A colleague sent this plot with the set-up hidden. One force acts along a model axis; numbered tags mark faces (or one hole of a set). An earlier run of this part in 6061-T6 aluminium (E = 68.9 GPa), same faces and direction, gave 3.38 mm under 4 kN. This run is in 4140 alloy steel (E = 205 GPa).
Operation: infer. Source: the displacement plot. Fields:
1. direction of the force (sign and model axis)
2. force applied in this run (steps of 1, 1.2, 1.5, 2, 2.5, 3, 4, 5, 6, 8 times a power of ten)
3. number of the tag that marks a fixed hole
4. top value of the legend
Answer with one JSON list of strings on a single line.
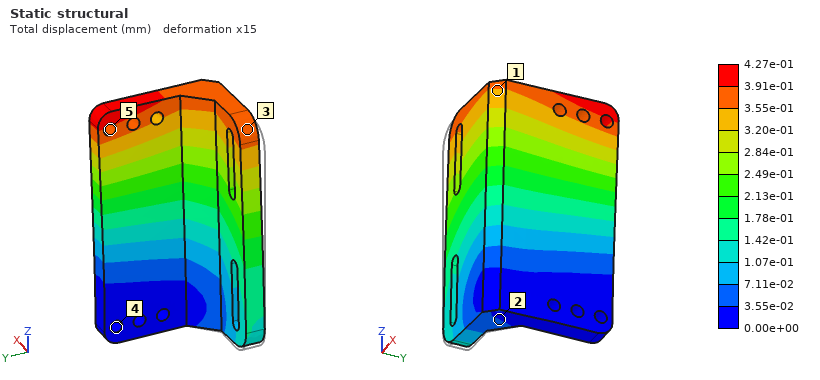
["+X", "1.5 kN", "4", "4.27e-01 mm"]
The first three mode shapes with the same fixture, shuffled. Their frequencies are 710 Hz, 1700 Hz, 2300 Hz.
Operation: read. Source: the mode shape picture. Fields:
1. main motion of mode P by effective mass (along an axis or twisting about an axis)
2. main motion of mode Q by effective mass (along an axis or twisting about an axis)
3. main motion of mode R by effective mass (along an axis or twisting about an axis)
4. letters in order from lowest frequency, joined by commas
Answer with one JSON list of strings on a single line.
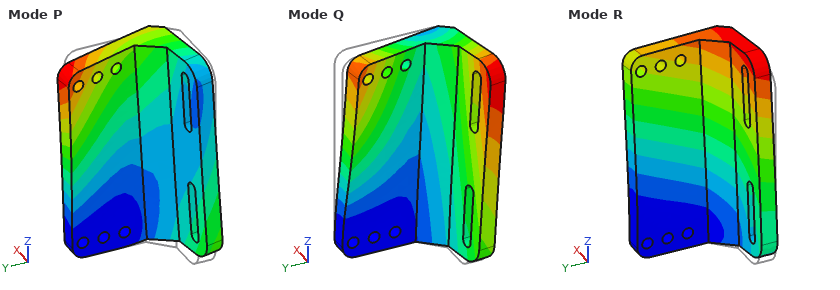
["along Y", "along Y", "along X", "R, Q, P"]
